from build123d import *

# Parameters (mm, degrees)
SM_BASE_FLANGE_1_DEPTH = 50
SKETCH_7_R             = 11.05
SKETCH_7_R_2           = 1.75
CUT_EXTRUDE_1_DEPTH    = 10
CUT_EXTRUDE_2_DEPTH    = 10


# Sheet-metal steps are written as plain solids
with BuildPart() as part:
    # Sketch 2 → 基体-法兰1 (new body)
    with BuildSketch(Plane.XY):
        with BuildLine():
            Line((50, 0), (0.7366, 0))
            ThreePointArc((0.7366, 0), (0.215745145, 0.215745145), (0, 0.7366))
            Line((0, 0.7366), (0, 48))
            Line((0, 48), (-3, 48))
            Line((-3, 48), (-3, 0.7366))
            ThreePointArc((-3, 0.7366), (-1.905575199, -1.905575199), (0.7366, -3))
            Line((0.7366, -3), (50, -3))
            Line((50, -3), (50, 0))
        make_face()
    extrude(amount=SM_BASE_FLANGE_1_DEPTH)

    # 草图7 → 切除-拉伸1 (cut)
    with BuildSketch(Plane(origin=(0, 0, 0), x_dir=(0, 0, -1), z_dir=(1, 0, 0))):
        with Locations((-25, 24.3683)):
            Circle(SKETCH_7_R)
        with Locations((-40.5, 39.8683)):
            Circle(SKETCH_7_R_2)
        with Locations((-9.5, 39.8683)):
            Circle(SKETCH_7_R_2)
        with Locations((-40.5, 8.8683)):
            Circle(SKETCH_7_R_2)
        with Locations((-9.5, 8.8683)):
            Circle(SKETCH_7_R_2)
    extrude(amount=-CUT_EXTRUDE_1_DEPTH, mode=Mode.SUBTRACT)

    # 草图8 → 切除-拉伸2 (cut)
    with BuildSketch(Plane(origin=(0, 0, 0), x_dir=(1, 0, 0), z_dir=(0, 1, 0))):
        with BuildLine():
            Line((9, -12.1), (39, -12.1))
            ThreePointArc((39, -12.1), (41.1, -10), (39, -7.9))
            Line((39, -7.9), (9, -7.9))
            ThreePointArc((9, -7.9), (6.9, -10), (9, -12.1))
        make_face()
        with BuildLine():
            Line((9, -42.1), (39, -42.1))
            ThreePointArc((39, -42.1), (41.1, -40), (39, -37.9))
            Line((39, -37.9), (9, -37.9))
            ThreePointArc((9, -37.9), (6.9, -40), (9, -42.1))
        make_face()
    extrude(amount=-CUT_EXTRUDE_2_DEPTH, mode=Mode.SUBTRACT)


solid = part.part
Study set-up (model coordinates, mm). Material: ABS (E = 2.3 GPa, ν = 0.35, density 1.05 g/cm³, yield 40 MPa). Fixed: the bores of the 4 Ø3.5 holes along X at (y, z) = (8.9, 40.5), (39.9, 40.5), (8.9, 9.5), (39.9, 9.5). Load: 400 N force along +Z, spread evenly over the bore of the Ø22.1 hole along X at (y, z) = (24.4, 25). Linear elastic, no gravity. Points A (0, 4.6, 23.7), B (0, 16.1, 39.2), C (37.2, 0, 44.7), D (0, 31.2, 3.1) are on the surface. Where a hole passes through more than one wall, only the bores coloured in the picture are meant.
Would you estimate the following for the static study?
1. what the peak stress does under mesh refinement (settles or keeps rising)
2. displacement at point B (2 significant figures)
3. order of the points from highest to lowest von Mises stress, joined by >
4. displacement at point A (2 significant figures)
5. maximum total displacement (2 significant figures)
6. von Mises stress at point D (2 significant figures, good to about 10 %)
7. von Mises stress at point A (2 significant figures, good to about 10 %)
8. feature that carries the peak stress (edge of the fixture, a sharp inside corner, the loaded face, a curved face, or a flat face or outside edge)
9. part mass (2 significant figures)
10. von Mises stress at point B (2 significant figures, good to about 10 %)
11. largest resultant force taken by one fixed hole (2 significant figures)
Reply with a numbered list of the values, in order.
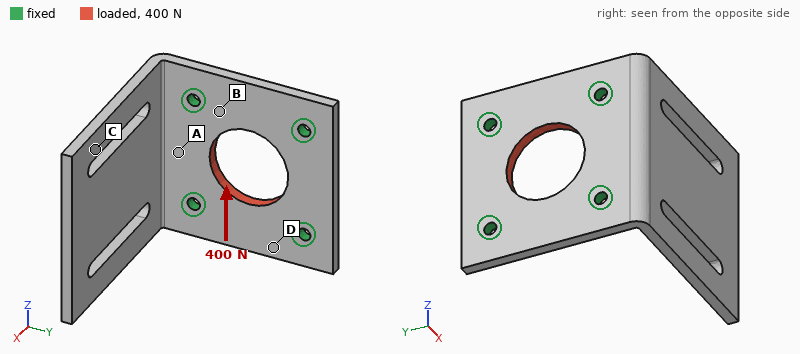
1. keeps rising
2. 15 µm
3. B > D > A > C
4. 5.2 µm
5. 28 µm
6. 1.5 MPa
7. 0.88 MPa
8. edge of the fixture
9. 14 g
10. 2.1 MPa
11. 100 N
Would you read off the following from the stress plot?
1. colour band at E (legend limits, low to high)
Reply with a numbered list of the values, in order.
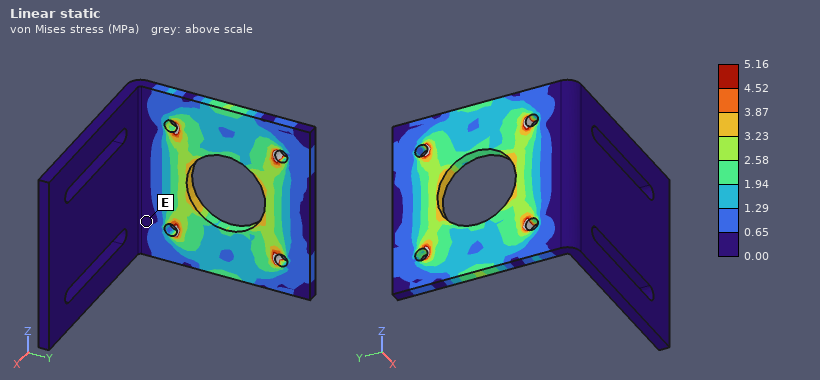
1. 0.00 to 0.65 MPa
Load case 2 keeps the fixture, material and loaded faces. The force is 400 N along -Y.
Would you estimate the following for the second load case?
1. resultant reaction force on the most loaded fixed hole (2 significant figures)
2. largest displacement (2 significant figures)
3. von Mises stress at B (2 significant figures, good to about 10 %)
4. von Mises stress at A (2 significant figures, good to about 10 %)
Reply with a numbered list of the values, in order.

1. 100 N
2. 30 µm
3. 2.5 MPa
4. 1.1 MPa
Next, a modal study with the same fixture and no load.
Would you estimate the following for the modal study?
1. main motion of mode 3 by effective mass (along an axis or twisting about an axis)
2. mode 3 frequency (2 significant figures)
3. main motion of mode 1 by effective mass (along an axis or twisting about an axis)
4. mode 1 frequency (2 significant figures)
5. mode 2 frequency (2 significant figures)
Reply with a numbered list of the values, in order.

1. along Z
2. 860 Hz
3. along Y
4. 210 Hz
5. 560 Hz
